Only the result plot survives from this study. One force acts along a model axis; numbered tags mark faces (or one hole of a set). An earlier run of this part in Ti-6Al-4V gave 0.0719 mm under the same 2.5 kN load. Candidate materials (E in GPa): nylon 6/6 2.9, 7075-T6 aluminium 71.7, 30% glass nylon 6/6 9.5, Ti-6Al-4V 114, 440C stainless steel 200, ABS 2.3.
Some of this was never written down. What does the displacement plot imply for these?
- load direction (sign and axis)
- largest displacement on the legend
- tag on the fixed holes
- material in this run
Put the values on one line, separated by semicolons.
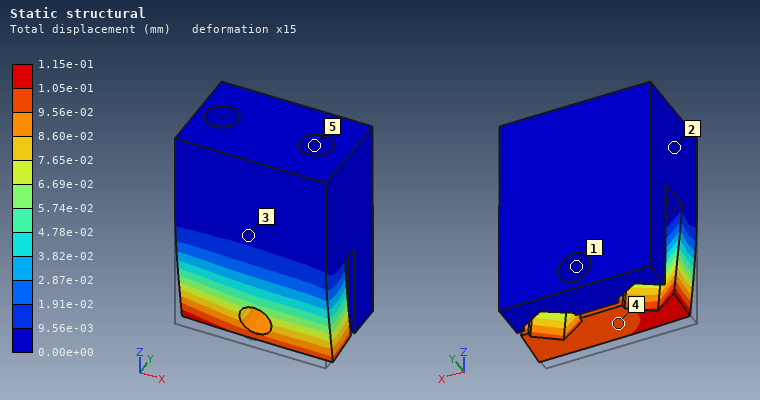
+Y; 1.15e-01 mm; 5; 7075-T6 aluminium
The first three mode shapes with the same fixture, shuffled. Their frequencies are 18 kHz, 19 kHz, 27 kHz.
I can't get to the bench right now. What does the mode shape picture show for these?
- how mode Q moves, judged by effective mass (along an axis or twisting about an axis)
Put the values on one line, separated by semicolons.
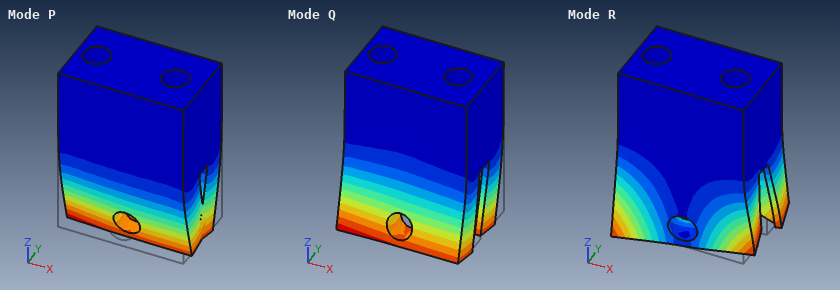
along Y
